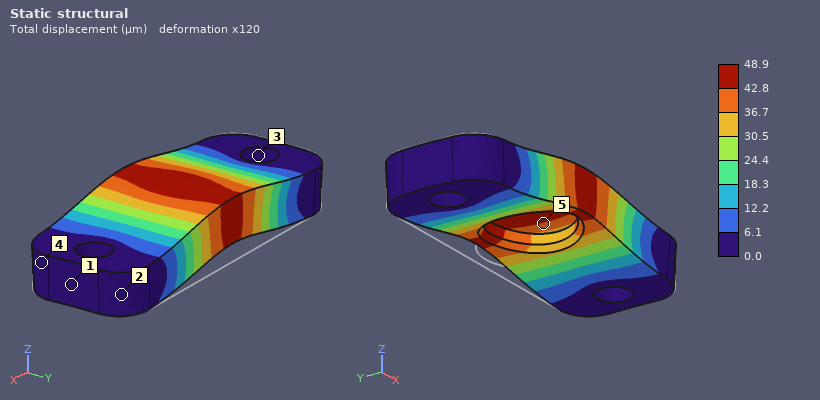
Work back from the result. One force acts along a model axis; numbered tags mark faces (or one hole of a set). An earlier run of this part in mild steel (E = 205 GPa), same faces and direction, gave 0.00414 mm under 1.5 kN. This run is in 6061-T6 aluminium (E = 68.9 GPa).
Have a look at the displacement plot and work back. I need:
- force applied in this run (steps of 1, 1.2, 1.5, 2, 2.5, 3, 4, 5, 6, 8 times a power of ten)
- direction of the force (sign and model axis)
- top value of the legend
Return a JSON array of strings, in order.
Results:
["6 kN", "+Z", "48.9 µm"]
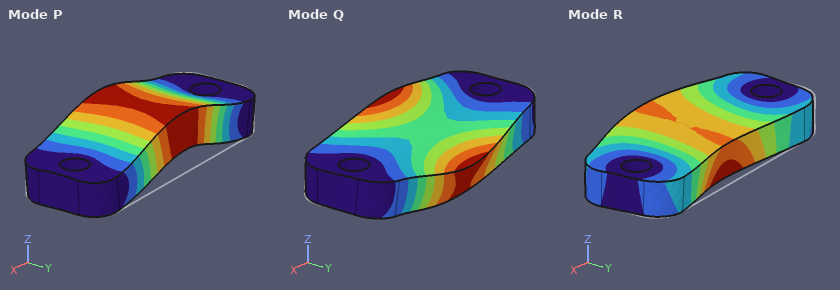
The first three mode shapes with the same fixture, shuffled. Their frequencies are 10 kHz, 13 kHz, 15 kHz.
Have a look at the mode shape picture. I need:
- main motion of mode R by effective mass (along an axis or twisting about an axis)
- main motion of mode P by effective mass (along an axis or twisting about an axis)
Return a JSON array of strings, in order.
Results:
["along Y", "along Z"]
